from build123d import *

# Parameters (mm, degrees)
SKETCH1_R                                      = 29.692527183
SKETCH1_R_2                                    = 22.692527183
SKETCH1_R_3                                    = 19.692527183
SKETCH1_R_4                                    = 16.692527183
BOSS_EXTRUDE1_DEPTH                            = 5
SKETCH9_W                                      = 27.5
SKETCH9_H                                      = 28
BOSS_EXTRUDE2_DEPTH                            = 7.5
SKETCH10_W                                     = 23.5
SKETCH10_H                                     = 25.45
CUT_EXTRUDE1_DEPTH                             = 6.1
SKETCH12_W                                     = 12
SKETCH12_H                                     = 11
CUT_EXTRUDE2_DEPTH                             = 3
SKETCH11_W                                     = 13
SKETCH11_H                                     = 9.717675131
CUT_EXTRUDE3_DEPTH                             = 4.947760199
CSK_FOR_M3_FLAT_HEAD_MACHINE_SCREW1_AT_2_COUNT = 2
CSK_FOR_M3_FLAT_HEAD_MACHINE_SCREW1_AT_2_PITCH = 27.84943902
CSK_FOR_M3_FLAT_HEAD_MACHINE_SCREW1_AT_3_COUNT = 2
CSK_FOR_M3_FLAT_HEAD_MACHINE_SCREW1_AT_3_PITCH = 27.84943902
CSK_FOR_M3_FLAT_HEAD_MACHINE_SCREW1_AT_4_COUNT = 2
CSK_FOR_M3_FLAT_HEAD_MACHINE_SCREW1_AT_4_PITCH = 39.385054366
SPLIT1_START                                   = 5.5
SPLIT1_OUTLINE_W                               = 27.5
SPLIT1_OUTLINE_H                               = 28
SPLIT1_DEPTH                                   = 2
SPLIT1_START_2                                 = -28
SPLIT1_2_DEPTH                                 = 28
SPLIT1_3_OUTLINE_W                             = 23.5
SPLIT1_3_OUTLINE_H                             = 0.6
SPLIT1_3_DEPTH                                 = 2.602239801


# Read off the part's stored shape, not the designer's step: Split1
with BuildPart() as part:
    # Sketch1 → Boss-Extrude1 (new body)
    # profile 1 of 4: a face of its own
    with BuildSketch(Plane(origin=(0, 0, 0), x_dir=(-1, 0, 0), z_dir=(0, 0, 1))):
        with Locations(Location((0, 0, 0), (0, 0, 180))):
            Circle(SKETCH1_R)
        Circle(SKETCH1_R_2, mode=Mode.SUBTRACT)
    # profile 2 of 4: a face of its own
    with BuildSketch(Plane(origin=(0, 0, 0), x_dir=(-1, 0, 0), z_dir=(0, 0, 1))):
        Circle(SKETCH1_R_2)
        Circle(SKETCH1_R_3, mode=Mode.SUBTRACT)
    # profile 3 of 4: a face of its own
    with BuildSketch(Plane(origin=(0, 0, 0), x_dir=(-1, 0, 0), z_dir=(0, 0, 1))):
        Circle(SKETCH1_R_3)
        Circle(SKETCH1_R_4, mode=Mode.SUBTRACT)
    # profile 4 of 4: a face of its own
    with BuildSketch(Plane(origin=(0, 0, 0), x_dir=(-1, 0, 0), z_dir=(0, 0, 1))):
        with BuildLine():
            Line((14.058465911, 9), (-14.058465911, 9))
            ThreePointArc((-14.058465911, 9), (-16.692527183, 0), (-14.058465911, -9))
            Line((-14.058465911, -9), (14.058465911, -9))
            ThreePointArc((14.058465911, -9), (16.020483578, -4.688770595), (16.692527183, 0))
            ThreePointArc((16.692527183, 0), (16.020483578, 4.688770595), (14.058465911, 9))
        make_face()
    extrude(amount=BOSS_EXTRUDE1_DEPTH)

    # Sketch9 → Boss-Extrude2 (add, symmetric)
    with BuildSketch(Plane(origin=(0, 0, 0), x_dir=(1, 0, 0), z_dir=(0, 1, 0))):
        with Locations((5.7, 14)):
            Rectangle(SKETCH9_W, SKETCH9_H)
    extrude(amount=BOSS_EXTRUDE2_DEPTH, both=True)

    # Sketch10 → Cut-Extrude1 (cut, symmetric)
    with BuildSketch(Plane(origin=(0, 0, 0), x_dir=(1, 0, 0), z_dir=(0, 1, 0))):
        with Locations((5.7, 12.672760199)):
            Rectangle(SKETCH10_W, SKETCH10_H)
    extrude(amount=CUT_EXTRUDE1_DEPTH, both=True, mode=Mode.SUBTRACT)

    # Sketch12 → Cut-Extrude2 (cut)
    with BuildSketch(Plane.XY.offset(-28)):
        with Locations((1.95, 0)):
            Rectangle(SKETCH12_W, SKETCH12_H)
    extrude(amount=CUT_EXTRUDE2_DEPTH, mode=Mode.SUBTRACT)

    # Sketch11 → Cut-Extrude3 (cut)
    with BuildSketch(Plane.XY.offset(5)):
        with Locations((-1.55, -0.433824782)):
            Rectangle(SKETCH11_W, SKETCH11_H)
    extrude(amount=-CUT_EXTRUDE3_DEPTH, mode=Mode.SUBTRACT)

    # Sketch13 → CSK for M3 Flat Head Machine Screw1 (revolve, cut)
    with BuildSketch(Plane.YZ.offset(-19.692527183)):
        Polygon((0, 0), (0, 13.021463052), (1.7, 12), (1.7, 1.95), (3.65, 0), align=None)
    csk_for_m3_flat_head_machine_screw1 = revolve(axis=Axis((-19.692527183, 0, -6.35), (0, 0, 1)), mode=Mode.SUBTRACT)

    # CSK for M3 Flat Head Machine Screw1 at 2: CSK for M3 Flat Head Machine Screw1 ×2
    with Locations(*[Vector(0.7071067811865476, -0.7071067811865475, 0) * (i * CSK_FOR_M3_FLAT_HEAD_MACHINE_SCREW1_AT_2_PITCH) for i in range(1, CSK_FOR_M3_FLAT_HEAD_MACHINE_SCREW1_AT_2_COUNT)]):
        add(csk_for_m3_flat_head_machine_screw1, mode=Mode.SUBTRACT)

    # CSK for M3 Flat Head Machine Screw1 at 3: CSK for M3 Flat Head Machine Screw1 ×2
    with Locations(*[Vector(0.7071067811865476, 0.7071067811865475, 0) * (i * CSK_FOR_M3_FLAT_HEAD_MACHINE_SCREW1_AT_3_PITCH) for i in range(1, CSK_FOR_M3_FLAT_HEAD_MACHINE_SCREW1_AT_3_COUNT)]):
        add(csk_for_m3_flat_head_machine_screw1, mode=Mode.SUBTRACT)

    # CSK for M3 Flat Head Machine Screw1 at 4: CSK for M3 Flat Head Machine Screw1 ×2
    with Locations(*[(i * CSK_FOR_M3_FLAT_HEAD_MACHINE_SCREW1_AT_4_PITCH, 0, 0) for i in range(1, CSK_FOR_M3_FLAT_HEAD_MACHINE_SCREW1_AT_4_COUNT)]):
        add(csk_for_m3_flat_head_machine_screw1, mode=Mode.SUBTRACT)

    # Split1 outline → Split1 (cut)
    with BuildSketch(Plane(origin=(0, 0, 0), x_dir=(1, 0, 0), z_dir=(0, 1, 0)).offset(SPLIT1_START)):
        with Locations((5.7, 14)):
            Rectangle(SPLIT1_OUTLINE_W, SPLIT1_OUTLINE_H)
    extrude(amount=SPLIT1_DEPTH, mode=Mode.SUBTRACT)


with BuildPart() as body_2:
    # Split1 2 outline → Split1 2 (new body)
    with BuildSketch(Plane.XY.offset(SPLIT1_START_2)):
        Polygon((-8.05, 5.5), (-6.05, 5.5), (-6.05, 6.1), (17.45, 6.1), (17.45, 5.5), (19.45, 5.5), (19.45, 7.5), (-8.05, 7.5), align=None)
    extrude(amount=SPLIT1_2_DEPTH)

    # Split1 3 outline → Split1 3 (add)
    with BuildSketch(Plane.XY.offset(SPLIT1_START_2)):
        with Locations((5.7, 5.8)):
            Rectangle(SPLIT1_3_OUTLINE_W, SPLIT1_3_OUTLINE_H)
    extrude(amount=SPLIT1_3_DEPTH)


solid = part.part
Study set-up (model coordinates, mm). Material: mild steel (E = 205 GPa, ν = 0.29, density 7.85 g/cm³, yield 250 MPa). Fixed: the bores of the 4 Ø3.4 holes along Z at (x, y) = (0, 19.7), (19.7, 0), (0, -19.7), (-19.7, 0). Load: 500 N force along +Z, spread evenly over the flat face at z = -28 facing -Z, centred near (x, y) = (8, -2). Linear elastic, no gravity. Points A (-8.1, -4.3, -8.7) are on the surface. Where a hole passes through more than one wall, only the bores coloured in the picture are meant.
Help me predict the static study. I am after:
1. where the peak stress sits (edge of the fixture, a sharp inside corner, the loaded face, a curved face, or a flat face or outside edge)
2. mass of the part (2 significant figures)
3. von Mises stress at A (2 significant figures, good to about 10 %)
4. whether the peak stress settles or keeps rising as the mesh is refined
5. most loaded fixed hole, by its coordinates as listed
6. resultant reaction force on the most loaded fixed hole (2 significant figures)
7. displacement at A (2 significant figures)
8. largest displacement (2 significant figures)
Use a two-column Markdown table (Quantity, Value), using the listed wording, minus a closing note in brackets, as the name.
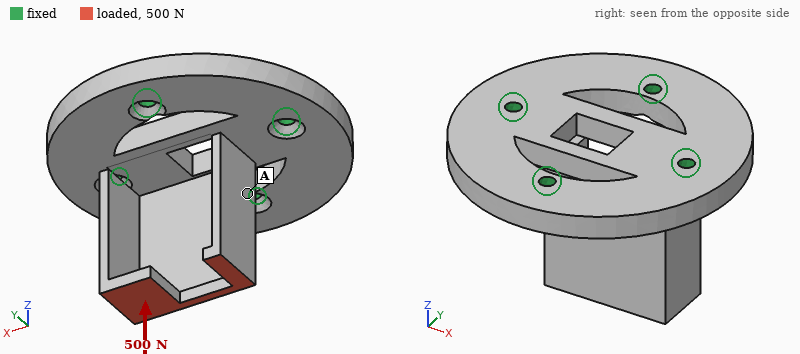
| Quantity | Value |
|---|---|
| where the peak stress sits | a sharp inside corner |
| mass of the part | 110 g |
| von Mises stress at A | 5.8 MPa |
| whether the peak stress settles or keeps rising as the mesh is refined | keeps rising |
| most loaded fixed hole, by its coordinates as listed | (19.7, 0) |
| resultant reaction force on the most loaded fixed hole | 320 N |
| displacement at A | 3.0 µm |
| largest displacement | 17 µm |
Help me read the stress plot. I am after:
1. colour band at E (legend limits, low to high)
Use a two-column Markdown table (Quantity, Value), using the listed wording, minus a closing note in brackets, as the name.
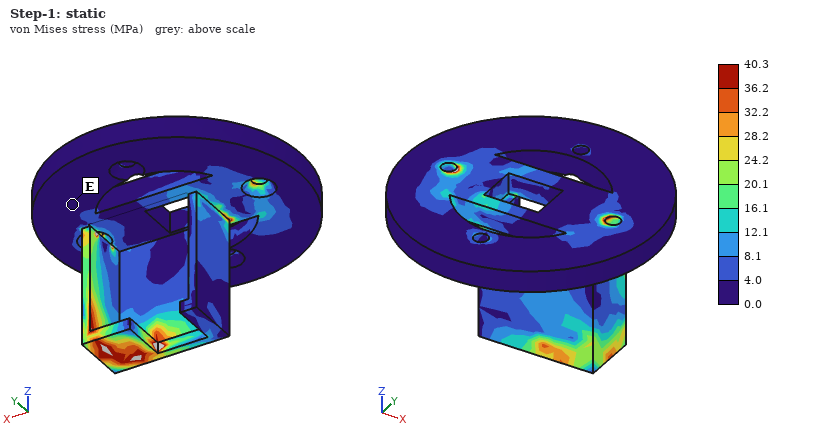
| Quantity | Value |
|---|---|
| colour band at E | 0.0 to 4.0 MPa |
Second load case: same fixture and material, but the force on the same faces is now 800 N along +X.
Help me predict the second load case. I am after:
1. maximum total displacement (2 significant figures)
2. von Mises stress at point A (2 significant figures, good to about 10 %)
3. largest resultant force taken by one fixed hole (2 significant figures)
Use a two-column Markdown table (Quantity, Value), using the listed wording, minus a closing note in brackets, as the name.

| Quantity | Value |
|---|---|
| maximum total displacement | 0.12 mm |
| von Mises stress at point A | 57 MPa |
| largest resultant force taken by one fixed hole | 780 N |
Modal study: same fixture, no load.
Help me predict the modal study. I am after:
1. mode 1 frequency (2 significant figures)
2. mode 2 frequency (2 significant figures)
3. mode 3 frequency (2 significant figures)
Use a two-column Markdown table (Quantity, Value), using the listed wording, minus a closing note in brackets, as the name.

| Quantity | Value |
|---|---|
| mode 1 frequency | 4400 Hz |
| mode 2 frequency | 5100 Hz |
| mode 3 frequency | 6600 Hz |
